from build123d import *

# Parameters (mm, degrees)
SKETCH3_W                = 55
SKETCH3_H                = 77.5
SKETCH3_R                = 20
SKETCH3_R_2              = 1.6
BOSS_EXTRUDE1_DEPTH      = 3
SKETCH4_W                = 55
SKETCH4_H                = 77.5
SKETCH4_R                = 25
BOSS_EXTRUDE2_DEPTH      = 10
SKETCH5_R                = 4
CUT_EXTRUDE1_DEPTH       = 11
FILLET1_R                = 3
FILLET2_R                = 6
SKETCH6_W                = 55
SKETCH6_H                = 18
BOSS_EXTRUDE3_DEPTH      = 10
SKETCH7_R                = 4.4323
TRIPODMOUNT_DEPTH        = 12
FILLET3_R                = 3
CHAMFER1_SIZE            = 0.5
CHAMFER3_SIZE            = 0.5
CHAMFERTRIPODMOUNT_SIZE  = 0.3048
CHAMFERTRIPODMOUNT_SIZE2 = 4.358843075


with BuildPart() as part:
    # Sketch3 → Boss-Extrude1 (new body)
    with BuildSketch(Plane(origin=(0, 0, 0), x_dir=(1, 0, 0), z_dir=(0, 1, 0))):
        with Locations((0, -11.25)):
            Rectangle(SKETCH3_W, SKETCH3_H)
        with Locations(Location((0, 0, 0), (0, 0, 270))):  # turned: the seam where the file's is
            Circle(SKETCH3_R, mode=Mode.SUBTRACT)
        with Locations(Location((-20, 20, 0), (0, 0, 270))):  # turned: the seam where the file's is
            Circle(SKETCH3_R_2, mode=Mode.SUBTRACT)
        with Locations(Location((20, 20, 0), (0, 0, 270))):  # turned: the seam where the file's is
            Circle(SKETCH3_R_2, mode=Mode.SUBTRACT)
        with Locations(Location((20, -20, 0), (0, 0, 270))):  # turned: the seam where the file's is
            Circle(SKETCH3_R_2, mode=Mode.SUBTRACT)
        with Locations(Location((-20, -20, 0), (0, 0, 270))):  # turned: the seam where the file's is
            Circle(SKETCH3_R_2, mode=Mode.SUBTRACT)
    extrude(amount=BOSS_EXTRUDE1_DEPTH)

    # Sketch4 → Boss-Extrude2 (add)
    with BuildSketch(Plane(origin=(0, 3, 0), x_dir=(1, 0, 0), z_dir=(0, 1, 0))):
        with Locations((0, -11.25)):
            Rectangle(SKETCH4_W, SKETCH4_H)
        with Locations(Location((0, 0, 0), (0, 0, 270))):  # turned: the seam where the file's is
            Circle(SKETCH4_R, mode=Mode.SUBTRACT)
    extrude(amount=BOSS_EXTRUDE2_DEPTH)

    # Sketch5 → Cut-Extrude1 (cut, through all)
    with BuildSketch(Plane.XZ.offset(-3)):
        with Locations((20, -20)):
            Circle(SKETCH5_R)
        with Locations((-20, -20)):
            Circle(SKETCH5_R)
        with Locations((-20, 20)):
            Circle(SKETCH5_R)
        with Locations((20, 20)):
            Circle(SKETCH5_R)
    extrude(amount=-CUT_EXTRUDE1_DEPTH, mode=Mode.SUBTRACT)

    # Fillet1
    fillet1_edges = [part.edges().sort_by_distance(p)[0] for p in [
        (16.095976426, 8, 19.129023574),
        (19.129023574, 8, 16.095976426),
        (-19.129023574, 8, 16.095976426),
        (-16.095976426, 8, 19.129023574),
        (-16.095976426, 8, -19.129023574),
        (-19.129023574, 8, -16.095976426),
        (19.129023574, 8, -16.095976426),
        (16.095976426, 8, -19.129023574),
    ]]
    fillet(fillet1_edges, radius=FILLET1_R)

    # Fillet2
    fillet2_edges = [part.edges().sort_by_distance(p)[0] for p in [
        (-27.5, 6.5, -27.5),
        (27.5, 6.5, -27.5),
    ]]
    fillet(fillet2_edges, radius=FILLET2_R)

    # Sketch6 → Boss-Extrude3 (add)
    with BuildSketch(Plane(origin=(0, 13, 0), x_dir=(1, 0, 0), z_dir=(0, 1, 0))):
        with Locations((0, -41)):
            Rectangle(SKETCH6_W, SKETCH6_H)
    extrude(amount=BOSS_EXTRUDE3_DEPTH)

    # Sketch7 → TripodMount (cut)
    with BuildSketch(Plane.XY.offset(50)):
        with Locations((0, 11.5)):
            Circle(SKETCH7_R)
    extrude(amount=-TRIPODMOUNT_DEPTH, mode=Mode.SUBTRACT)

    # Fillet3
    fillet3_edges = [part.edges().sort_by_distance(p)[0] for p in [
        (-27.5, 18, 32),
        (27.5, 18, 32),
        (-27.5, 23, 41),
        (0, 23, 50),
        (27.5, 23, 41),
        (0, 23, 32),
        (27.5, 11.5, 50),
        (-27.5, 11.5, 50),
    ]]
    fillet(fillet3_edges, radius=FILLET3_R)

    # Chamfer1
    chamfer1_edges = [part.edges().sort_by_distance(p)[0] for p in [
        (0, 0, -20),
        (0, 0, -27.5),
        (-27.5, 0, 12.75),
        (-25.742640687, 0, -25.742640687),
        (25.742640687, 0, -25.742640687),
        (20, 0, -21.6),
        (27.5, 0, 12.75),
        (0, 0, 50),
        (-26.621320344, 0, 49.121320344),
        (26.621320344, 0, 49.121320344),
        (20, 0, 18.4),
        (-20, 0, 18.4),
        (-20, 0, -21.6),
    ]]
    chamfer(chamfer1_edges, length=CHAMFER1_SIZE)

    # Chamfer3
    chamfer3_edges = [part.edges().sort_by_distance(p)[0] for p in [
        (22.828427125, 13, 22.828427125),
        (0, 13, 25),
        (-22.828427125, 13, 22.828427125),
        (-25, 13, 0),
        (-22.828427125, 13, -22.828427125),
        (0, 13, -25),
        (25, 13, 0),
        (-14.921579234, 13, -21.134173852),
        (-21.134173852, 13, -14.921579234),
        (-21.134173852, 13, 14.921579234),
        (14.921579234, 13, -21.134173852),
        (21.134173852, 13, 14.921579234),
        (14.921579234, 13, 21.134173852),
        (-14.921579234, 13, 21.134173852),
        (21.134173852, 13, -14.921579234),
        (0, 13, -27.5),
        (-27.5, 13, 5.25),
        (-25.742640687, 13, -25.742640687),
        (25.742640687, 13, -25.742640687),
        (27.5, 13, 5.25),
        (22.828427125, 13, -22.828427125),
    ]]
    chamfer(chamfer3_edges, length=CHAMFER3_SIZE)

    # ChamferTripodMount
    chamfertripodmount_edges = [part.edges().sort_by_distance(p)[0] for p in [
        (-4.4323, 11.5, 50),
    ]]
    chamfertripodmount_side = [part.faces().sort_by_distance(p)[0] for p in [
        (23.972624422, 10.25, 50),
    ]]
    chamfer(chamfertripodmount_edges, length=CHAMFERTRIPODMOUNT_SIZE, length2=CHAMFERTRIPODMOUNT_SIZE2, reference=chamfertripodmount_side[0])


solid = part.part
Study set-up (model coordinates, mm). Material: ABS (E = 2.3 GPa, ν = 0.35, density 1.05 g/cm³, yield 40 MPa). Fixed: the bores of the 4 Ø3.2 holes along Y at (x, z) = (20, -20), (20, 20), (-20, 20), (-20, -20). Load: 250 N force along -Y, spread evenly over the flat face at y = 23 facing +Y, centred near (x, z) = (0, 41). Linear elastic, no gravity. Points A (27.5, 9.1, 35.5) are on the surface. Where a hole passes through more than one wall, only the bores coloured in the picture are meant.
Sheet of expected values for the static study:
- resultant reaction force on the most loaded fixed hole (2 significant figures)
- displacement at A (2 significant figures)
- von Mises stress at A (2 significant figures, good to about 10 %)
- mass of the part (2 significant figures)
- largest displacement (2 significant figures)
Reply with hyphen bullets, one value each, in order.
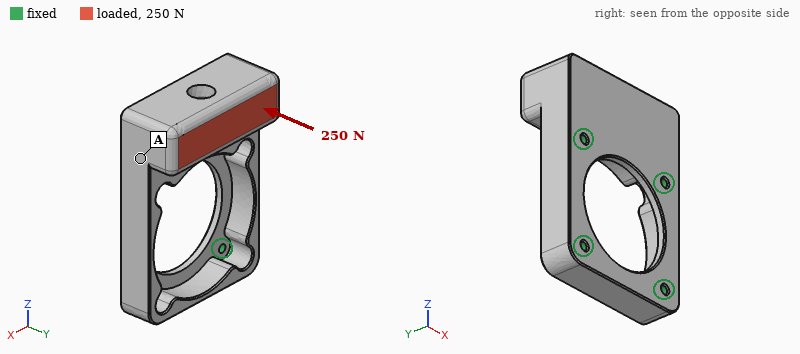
- 210 N
- 0.31 mm
- 2.8 MPa
- 40 g
- 0.68 mm
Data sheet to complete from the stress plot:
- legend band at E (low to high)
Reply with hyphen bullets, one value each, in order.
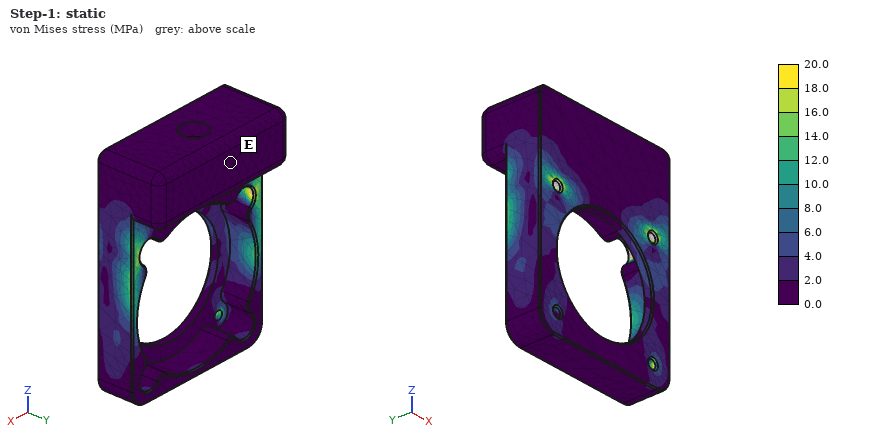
- 0.0 to 2.0 MPa
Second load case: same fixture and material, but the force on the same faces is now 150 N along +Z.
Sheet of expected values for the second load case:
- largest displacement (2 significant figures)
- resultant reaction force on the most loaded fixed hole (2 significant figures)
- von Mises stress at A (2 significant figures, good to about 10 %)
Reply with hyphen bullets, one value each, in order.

- 0.43 mm
- 79 N
- 1.9 MPa
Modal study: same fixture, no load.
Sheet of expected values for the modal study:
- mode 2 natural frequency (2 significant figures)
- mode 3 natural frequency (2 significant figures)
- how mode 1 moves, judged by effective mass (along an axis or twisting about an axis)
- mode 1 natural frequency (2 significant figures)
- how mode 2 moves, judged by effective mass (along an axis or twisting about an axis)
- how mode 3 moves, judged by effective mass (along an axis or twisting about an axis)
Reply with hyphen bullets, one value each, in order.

- 2000 Hz
- 2800 Hz
- along Y
- 700 Hz
- along X
- along X
